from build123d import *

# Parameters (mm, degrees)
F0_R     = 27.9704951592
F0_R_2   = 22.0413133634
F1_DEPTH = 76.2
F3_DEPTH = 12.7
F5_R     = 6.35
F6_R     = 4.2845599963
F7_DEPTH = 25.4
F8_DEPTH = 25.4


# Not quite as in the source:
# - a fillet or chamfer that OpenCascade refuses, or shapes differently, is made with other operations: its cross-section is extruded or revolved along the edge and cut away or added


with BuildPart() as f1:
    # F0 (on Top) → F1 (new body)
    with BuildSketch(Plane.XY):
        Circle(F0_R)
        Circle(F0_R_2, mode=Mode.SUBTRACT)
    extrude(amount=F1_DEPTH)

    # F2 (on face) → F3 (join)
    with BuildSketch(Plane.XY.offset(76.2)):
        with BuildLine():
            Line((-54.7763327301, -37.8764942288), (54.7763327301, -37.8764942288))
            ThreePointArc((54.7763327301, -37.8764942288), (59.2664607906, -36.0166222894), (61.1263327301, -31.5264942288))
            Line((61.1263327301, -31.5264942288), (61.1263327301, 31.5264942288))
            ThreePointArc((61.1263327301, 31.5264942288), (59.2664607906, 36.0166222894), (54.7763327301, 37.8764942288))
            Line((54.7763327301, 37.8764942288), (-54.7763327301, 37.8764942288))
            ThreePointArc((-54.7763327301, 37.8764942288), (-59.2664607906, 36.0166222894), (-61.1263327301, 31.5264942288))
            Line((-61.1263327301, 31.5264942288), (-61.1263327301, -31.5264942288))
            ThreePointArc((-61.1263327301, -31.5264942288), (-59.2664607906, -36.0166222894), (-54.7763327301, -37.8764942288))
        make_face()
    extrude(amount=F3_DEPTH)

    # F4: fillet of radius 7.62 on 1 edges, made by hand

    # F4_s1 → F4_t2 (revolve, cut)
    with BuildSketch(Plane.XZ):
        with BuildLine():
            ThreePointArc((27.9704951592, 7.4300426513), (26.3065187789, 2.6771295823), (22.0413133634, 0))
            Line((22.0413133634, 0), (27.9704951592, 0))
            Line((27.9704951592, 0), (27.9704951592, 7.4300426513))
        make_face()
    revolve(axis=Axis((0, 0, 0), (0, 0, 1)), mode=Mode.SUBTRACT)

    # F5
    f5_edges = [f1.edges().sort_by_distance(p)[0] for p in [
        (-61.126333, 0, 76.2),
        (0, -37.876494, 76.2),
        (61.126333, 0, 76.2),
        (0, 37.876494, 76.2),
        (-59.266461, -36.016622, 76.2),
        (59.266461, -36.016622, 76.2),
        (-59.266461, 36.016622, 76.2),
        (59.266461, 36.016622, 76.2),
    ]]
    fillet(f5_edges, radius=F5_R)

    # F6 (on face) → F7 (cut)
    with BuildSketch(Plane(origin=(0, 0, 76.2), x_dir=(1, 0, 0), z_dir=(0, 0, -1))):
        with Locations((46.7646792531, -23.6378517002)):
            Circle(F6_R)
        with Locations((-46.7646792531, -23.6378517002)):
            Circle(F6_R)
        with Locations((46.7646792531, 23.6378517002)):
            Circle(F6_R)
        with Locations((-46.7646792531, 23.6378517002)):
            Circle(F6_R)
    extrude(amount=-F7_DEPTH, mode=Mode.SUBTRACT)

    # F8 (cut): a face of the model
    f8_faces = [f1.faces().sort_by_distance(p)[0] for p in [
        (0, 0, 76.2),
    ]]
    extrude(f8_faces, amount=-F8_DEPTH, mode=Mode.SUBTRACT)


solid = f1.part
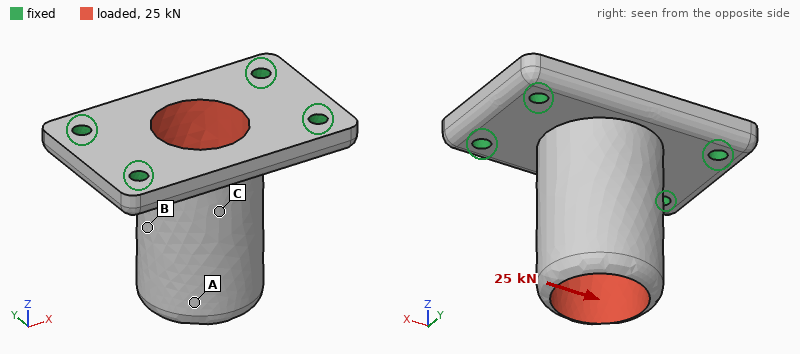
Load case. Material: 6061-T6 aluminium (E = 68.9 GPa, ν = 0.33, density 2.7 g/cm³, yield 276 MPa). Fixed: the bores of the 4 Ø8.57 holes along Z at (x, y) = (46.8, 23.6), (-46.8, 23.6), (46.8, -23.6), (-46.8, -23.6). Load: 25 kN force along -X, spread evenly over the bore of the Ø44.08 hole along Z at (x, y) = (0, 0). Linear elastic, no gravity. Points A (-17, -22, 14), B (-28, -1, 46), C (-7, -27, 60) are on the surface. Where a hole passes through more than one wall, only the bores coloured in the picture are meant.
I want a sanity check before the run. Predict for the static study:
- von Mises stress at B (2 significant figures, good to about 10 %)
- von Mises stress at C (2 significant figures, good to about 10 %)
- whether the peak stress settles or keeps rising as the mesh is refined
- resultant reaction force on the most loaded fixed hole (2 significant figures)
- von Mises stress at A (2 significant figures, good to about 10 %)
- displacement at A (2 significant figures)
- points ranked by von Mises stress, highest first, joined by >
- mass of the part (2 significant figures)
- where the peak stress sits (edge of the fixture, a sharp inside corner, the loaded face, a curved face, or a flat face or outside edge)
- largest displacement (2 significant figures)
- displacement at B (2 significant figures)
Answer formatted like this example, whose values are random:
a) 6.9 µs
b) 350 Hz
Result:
a) 25 MPa
b) 43 MPa
c) keeps rising
d) 9.4 kN
e) 12 MPa
f) 0.26 mm
g) C > B > A
h) 430 g
i) edge of the fixture
j) 0.32 mm
k) 0.17 mm
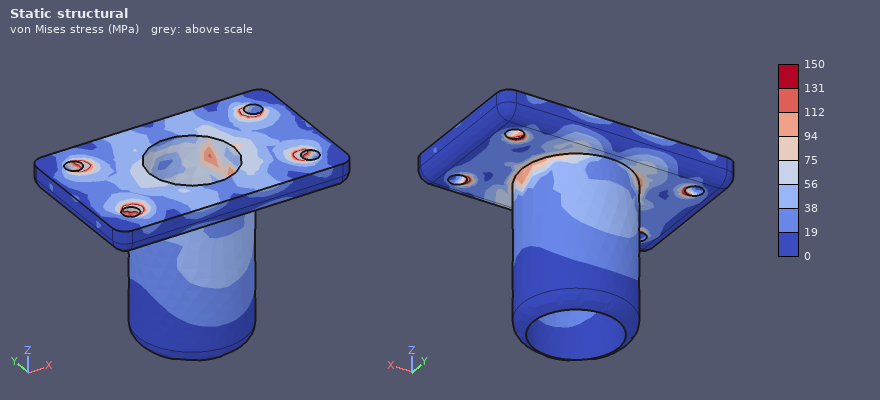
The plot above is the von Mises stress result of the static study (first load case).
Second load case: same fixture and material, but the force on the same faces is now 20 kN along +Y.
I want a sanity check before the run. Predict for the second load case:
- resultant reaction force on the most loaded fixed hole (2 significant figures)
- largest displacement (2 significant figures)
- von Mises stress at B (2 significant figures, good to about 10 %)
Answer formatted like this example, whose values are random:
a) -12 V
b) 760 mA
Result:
a) 9.9 kN
b) 0.48 mm
c) 31 MPa
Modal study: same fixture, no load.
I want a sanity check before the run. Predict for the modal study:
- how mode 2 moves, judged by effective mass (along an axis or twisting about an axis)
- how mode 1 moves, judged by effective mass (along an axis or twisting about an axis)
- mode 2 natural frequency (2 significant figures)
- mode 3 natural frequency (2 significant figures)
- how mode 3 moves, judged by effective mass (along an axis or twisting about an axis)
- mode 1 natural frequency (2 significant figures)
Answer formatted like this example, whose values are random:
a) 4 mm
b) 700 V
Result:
a) along X
b) along Y
c) 3600 Hz
d) 5300 Hz
e) along Z
f) 2600 Hz
